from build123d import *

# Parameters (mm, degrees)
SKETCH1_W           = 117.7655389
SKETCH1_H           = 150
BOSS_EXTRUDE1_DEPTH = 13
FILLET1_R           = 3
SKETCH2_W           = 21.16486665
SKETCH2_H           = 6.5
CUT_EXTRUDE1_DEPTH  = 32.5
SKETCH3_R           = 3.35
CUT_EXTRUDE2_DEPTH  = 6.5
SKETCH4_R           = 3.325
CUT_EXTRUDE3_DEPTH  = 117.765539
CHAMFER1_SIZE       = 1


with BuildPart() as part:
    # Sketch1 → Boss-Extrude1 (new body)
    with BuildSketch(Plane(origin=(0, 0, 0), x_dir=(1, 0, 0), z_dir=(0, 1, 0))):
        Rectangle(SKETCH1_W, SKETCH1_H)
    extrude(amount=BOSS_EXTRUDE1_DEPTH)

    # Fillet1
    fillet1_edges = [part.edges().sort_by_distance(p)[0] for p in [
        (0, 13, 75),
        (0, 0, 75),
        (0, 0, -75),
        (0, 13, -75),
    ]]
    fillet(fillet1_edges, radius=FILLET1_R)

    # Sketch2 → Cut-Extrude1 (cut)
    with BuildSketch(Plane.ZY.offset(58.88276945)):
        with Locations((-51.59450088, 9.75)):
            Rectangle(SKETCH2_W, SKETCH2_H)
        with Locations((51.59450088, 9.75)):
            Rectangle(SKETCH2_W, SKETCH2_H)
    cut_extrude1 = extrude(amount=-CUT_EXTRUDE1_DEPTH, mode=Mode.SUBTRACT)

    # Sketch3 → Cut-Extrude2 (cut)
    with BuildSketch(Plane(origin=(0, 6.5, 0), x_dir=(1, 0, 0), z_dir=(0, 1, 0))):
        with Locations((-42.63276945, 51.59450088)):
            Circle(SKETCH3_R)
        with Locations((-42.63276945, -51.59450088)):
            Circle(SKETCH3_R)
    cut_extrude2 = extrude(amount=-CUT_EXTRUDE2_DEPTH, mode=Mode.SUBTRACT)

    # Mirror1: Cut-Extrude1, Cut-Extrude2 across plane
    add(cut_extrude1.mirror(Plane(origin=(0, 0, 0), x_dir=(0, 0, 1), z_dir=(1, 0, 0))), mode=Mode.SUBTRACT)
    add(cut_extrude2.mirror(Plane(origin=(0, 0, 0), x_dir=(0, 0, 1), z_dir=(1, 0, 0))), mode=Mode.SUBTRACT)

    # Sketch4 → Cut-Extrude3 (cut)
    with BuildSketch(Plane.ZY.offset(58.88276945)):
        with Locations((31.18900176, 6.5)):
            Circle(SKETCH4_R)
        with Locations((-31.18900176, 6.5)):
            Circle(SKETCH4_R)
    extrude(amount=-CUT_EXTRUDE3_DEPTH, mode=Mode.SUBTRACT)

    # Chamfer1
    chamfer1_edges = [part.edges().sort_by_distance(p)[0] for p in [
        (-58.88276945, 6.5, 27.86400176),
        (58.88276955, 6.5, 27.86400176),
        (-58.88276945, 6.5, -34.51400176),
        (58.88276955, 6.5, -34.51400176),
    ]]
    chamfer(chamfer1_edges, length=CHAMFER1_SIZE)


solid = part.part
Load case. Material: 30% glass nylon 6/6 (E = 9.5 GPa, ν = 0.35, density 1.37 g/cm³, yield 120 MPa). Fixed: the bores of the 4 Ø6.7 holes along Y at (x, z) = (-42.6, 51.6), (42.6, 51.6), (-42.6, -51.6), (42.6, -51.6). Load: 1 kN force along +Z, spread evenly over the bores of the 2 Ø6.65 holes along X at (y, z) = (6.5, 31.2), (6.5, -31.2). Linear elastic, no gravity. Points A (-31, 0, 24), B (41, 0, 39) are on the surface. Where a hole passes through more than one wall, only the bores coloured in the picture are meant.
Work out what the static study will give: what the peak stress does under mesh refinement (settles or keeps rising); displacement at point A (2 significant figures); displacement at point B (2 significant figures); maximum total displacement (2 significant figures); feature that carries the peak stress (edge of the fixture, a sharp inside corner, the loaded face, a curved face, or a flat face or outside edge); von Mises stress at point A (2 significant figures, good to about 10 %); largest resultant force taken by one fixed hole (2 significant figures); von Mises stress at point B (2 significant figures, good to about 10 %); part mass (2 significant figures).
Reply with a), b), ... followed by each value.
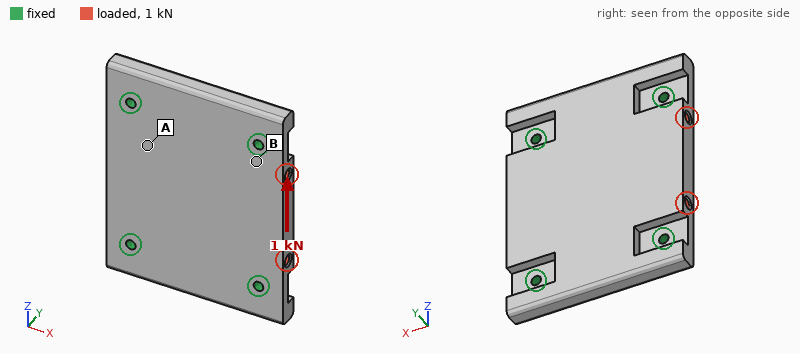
a) keeps rising
b) 3.3 µm
c) 1.5 µm
d) 4.7 µm
e) edge of the fixture
f) 0.48 MPa
g) 250 N
h) 1.2 MPa
i) 280 g
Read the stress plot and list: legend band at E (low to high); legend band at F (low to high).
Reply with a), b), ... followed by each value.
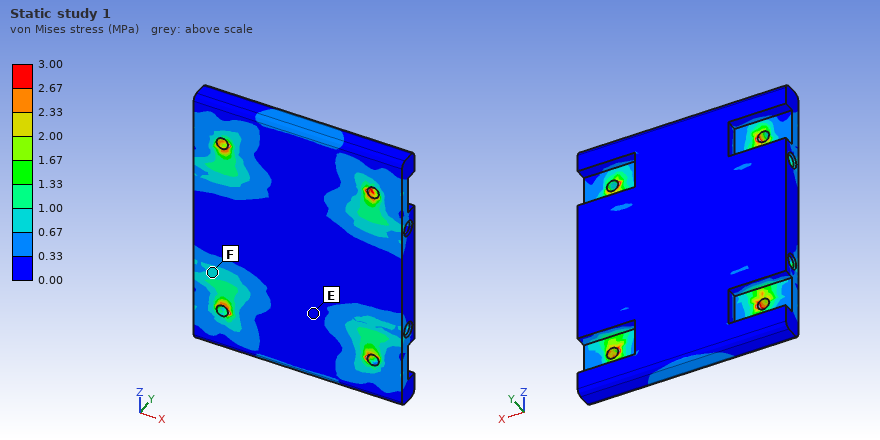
a) 0.00 to 0.33 MPa
b) 0.67 to 1.00 MPa
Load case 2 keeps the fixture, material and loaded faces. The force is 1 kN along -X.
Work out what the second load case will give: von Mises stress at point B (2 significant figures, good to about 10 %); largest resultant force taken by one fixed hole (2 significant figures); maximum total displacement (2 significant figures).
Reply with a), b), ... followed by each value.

a) 0.82 MPa
b) 260 N
c) 5.6 µm
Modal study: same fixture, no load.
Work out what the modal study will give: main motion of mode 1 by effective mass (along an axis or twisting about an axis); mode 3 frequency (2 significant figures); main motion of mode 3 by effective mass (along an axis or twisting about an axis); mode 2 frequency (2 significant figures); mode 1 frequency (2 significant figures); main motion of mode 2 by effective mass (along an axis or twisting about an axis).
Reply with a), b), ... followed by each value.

a) along Y
b) 2600 Hz
c) along Y
d) 2500 Hz
e) 1800 Hz
f) twisting about Z
